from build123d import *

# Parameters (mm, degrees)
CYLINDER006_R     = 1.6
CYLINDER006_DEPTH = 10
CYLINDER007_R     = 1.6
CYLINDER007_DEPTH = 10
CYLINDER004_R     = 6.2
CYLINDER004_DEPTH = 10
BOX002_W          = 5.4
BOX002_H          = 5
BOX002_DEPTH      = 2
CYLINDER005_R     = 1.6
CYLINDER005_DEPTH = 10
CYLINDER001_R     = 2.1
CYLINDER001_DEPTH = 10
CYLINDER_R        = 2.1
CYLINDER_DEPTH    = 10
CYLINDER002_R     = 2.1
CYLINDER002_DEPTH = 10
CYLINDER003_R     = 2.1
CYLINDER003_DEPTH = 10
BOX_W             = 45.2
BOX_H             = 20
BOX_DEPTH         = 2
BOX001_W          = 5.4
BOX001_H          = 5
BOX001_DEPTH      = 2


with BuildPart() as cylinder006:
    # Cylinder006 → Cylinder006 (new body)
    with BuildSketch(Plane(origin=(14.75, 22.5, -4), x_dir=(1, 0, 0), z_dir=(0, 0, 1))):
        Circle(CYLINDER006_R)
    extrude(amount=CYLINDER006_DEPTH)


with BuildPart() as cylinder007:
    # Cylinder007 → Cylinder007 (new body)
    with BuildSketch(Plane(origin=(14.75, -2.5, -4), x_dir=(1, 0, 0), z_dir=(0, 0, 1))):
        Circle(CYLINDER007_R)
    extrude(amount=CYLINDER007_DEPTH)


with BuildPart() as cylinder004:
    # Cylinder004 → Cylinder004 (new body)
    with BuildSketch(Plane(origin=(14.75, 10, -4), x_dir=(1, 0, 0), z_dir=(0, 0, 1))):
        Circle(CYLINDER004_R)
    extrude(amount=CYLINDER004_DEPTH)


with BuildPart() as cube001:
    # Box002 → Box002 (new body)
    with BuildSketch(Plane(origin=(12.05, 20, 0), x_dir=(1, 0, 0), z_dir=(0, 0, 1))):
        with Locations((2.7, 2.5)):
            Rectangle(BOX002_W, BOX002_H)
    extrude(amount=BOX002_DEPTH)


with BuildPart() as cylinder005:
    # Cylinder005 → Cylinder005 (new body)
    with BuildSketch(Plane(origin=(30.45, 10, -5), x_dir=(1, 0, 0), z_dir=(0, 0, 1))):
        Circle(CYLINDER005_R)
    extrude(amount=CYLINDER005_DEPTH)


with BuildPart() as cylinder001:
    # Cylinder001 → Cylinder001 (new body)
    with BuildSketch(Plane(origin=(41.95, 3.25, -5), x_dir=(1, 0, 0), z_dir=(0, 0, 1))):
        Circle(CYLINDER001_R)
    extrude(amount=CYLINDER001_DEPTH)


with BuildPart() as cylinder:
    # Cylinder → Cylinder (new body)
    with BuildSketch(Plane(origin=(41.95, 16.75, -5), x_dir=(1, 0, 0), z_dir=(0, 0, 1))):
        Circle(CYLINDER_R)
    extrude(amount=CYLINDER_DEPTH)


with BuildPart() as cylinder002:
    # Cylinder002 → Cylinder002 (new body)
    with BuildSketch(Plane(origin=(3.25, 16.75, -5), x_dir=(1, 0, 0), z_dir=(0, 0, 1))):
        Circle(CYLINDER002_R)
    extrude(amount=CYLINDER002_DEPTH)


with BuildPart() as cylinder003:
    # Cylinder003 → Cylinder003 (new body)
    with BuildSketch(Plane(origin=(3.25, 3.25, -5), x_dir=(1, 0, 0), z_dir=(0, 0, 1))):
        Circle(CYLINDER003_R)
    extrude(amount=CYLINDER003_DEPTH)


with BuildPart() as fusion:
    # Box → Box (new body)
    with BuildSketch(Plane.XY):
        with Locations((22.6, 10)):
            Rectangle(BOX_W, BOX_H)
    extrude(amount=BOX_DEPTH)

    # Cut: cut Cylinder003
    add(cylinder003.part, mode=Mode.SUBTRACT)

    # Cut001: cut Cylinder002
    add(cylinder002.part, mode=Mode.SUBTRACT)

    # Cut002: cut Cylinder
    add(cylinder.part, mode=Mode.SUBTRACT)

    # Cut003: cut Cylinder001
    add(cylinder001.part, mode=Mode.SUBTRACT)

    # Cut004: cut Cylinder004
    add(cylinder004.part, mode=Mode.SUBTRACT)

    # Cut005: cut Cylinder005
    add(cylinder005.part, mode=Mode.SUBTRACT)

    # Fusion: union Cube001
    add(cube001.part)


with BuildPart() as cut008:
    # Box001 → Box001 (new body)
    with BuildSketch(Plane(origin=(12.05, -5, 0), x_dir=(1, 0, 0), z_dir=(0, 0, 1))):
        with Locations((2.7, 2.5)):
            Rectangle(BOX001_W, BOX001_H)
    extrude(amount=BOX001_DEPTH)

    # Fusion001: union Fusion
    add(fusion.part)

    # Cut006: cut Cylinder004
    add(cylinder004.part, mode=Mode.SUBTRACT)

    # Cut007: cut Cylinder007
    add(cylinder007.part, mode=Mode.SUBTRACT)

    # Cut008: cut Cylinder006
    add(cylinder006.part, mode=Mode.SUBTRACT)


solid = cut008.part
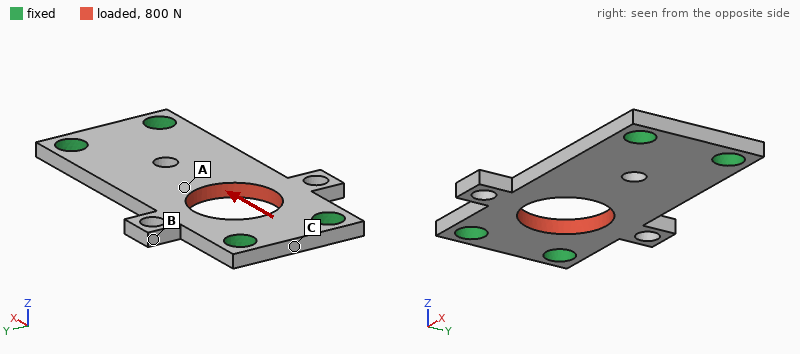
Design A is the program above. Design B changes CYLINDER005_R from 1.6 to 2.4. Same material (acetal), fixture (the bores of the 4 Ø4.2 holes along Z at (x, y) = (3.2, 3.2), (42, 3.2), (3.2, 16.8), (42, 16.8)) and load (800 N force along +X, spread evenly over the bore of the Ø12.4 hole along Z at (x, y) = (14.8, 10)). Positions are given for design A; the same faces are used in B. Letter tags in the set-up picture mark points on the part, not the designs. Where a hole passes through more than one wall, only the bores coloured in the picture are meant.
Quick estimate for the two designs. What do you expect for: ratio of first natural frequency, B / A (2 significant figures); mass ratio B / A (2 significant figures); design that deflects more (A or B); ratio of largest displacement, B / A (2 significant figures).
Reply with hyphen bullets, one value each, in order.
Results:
- 1.0
- 0.99
- B
- 1.1
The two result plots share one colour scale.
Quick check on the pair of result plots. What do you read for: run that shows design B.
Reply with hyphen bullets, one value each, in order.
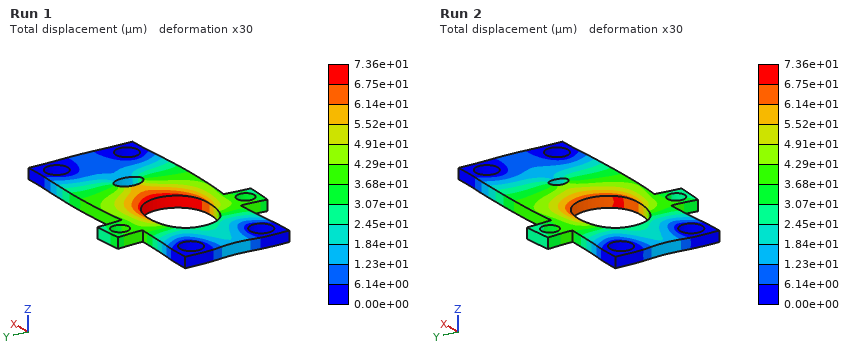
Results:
- Run 1
